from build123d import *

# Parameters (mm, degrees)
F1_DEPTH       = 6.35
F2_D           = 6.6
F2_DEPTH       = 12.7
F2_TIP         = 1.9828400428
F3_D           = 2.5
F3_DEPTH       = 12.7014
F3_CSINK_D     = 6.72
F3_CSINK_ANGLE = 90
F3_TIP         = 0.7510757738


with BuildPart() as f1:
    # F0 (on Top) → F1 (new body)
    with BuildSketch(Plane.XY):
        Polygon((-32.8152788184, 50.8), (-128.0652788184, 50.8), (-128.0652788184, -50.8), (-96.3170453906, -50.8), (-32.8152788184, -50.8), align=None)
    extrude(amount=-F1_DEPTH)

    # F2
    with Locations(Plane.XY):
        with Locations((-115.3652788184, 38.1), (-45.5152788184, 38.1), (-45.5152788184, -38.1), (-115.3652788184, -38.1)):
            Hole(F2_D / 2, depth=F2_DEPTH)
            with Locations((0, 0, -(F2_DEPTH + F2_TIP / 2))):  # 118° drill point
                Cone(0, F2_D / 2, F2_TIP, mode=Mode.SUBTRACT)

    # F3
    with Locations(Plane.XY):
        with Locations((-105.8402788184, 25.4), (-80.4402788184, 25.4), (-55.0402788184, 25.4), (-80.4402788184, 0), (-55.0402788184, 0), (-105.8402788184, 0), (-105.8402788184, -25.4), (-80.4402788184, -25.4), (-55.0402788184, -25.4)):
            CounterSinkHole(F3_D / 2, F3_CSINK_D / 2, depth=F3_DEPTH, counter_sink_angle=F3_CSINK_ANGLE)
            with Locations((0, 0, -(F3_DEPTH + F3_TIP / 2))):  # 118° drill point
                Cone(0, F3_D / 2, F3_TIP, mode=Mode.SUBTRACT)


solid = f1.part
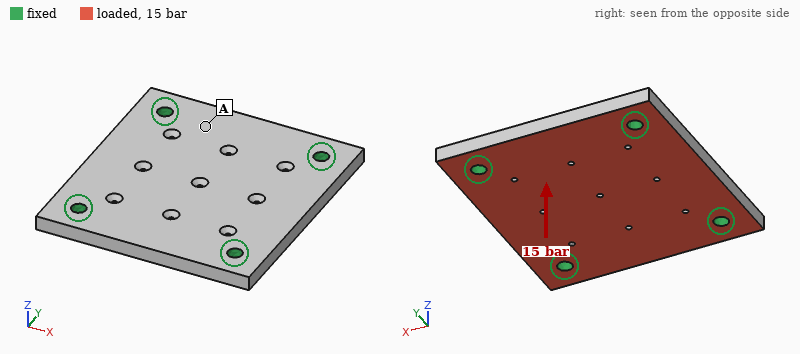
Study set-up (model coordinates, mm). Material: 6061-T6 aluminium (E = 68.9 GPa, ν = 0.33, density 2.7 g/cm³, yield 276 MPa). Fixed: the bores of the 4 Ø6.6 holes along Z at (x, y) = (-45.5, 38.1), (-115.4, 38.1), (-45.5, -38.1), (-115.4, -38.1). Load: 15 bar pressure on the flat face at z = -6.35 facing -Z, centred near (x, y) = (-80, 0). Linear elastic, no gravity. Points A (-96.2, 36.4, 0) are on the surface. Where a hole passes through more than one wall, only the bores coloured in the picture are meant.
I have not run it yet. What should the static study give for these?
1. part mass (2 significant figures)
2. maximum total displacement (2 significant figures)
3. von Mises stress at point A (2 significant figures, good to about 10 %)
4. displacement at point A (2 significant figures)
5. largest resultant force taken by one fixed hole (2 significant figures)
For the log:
160 g
0.19 mm
35 MPa
0.063 mm
3.6 kN
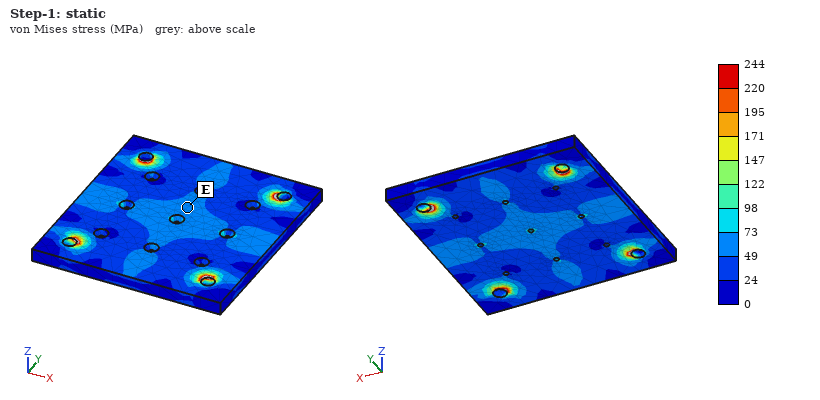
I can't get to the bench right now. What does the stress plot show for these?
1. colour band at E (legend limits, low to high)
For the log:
49 to 73 MPa
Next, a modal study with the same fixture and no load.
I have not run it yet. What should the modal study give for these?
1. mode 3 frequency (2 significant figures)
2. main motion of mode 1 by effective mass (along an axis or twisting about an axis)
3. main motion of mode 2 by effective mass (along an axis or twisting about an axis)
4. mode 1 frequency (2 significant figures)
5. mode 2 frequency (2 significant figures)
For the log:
6700 Hz
along Z
twisting about Y
4300 Hz
6200 Hz
